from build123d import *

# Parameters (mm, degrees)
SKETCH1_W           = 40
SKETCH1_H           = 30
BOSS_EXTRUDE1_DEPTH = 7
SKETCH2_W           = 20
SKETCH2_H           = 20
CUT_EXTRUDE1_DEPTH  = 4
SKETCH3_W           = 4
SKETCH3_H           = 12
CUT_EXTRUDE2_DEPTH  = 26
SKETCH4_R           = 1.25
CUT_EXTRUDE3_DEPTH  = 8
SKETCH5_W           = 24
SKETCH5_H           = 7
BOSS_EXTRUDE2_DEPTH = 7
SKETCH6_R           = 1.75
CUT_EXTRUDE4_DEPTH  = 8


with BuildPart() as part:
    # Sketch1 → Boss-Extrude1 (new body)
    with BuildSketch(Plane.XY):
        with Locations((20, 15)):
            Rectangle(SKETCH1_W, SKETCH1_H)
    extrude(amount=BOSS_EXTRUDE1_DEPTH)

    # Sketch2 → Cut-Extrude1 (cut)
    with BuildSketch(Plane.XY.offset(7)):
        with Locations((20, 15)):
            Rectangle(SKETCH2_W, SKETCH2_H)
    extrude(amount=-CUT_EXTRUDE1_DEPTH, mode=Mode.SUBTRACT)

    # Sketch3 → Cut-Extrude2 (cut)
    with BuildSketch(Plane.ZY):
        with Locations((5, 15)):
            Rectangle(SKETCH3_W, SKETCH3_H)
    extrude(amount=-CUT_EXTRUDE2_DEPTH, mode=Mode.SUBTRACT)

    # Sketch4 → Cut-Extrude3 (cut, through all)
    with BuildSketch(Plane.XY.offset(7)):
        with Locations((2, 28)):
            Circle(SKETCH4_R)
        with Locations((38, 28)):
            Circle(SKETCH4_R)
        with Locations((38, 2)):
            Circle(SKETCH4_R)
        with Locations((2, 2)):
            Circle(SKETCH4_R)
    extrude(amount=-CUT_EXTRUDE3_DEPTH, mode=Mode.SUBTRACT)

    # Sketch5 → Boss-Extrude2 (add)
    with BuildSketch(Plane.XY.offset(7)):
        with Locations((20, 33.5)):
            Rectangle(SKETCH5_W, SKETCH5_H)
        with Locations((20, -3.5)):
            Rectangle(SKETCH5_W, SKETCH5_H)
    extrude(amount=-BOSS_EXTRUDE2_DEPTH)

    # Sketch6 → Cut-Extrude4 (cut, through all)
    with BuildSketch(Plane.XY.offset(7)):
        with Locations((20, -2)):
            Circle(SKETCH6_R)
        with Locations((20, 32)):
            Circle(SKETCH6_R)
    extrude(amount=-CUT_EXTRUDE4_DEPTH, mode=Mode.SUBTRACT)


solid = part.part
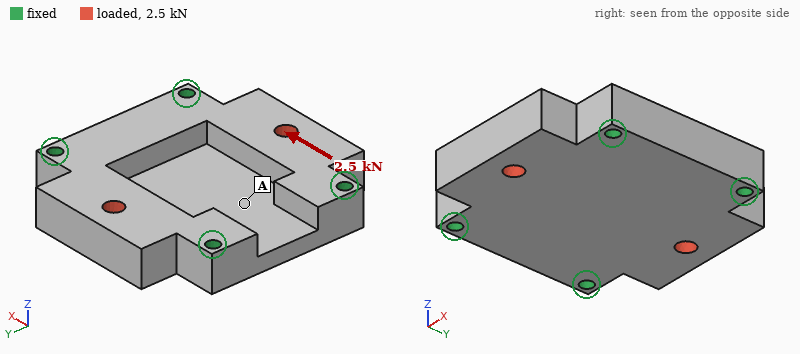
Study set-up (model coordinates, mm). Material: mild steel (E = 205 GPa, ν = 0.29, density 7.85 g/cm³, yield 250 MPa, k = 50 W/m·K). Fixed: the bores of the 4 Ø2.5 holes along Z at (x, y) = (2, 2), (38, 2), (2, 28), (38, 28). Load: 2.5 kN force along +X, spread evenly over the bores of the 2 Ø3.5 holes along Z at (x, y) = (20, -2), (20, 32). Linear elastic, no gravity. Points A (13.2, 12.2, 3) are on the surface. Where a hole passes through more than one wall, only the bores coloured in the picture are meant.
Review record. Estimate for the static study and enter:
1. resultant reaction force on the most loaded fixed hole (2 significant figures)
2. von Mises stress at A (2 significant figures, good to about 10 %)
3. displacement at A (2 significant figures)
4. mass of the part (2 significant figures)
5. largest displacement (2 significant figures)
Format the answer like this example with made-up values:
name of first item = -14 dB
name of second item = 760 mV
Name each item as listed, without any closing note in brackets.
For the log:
resultant reaction force on the most loaded fixed hole = 630 N
von Mises stress at A = 5.1 MPa
displacement at A = 0.54 µm
mass of the part = 66 g
largest displacement = 1.6 µm
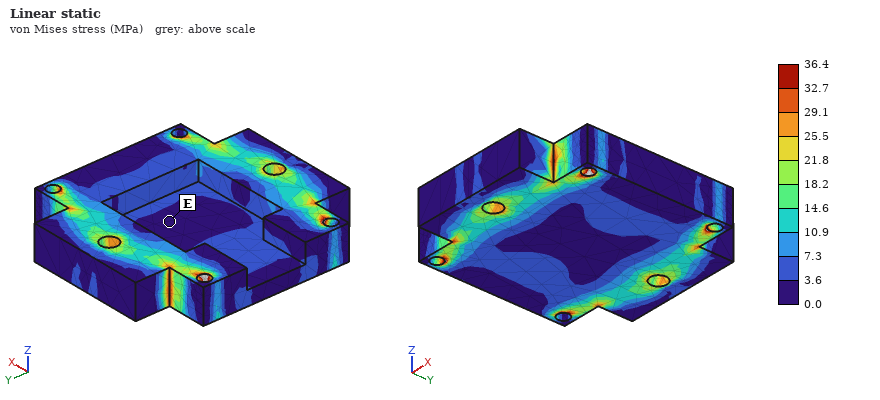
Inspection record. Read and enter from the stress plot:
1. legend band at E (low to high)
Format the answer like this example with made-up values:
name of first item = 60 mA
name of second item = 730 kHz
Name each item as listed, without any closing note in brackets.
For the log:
legend band at E = 0.0 to 3.6 MPa
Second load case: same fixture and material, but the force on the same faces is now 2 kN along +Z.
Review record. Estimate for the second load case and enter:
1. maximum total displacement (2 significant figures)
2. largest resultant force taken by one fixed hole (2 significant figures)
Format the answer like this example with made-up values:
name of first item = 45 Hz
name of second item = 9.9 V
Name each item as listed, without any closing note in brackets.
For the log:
maximum total displacement = 13 µm
largest resultant force taken by one fixed hole = 530 N
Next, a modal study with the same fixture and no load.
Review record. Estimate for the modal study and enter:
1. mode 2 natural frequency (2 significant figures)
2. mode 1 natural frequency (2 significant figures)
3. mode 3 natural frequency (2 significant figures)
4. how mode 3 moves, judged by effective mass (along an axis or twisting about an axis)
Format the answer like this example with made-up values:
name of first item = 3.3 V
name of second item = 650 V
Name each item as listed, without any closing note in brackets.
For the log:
mode 2 natural frequency = 16 kHz
mode 1 natural frequency = 15 kHz
mode 3 natural frequency = 21 kHz
how mode 3 moves, judged by effective mass = along Z
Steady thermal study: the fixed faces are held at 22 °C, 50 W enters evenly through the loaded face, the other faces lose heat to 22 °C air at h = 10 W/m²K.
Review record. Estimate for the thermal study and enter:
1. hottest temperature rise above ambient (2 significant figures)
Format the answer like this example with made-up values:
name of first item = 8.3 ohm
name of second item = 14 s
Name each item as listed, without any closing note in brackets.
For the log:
hottest temperature rise above ambient = 72 K
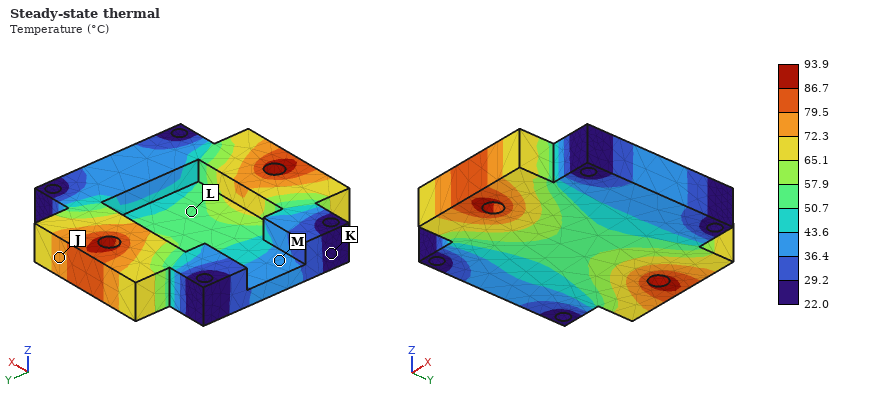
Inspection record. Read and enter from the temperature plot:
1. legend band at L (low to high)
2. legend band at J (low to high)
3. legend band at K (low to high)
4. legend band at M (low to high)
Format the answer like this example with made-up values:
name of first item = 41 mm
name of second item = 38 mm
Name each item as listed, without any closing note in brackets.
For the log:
legend band at L = 50.7 to 57.9 °C
legend band at J = 72.3 to 79.5 °C
legend band at K = 22.0 to 29.2 °C
legend band at M = 36.4 to 43.6 °C
